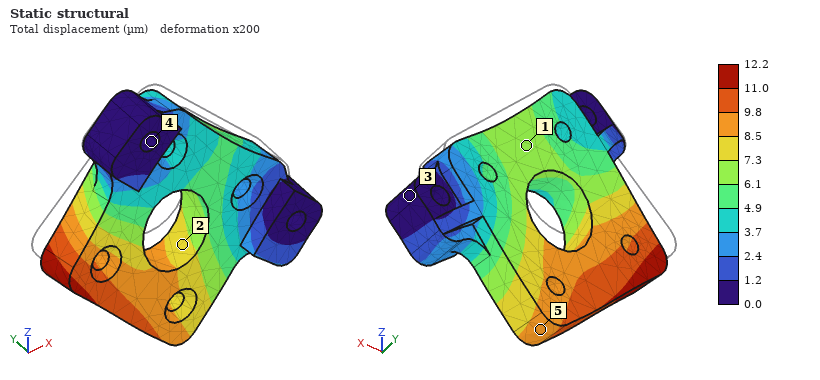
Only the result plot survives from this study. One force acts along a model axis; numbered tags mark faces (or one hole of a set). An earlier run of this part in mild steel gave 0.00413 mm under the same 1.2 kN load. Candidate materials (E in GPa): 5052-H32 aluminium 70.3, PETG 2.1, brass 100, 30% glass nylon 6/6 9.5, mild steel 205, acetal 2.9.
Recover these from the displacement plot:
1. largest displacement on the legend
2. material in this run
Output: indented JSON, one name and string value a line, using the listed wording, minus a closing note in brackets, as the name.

{
  "largest displacement on the legend": "12.2 µm",
  "material in this run": "5052-H32 aluminium"
}
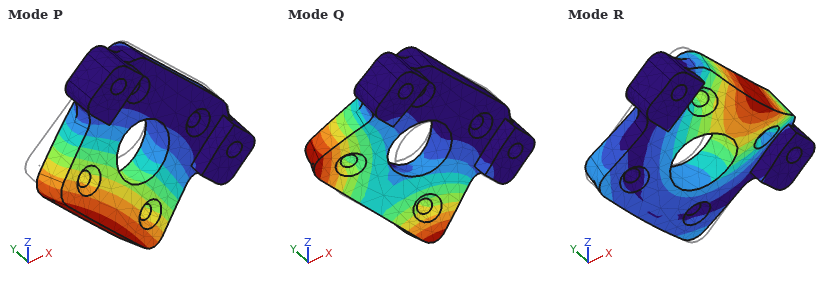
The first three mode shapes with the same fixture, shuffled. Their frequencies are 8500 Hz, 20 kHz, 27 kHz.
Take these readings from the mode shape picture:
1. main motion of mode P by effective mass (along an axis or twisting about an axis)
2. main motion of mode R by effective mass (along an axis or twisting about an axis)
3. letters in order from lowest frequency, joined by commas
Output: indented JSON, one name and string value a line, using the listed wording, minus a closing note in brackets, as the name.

{
  "main motion of mode P by effective mass": "along Y",
  "main motion of mode R by effective mass": "along Y",
  "letters in order from lowest frequency, joined by commas": "P, Q, R"
}
